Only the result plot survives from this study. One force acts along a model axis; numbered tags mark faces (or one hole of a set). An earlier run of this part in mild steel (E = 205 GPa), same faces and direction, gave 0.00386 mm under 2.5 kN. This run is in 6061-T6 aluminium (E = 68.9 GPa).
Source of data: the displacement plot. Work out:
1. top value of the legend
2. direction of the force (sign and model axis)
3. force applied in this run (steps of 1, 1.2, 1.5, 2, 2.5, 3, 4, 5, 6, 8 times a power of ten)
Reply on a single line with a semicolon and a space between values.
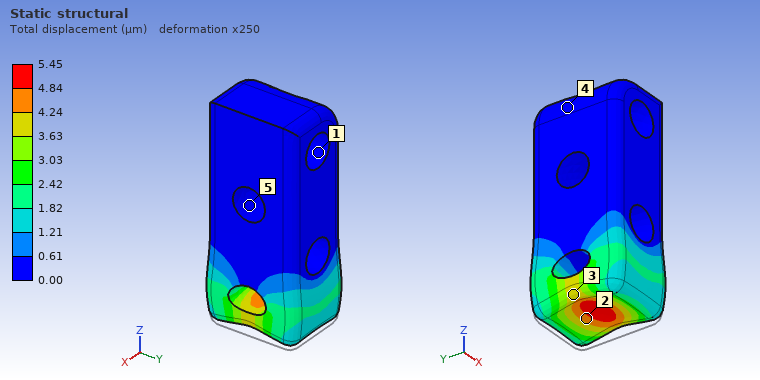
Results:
5.45 µm; +Z; 1.2 kN
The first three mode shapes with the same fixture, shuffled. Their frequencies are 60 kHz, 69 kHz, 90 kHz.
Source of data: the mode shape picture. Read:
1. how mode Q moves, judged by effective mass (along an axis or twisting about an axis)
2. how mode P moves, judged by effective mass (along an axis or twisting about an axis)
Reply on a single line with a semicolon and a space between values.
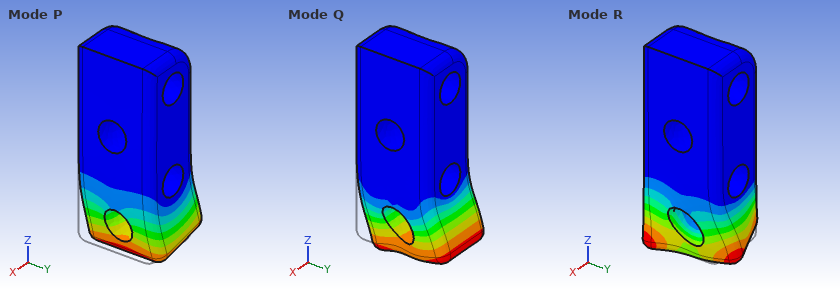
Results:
along Y; along X
